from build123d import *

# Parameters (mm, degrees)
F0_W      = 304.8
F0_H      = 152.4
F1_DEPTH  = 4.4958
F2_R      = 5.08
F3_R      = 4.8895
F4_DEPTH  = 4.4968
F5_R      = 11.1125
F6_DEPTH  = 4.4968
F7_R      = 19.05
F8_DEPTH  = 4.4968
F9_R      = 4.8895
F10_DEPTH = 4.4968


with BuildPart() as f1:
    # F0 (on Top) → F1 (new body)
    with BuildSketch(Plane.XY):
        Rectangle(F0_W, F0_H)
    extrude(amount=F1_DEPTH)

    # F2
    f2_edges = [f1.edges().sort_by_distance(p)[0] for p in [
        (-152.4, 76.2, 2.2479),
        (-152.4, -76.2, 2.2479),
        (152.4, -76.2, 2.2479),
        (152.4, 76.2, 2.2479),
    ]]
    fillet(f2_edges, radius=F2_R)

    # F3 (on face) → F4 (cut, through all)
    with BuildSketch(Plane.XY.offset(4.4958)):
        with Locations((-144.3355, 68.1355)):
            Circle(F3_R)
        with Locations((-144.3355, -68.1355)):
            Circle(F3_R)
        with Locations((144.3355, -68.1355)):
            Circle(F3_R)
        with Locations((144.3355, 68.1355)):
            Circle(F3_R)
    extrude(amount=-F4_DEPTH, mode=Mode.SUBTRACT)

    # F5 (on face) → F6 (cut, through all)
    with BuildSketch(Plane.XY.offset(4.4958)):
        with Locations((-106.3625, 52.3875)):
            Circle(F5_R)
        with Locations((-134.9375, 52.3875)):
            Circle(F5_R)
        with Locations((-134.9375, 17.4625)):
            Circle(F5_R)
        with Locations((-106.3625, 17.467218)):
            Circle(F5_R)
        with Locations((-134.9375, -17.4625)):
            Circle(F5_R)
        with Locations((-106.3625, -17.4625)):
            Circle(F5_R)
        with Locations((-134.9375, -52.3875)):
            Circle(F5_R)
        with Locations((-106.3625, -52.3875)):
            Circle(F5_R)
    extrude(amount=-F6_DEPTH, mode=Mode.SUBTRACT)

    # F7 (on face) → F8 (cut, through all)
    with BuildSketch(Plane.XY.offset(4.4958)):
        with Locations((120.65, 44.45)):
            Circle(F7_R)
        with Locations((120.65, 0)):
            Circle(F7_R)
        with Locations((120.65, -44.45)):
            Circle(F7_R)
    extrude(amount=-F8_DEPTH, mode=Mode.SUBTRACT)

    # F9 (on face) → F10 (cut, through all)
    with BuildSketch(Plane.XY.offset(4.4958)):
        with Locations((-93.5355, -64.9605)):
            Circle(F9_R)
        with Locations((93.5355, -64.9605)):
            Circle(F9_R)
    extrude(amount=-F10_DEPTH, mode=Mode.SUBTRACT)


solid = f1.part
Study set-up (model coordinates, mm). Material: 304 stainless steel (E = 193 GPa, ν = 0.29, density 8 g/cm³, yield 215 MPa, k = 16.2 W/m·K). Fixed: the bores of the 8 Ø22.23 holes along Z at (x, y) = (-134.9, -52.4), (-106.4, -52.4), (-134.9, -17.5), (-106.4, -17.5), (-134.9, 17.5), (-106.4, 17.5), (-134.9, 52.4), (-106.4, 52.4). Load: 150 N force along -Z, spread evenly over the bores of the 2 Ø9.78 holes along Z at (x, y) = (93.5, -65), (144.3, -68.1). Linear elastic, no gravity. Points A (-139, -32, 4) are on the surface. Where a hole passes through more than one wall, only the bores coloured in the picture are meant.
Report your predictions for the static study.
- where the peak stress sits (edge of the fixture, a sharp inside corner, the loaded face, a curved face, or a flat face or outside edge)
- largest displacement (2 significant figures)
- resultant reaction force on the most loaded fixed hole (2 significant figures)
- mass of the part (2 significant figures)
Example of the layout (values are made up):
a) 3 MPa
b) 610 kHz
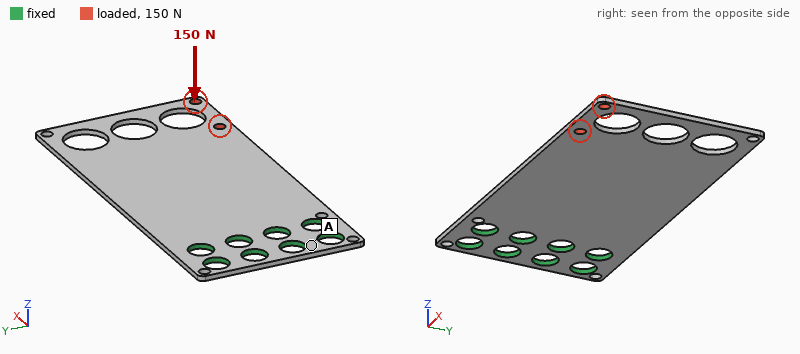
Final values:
a) a curved face
b) 3.2 mm
c) 91 N
d) 1.4 kg
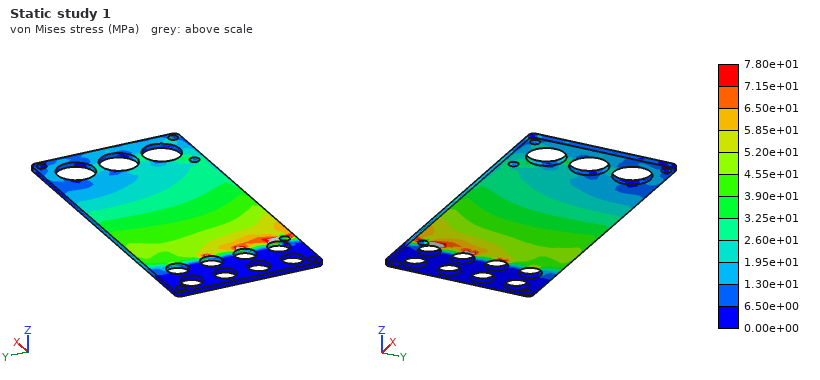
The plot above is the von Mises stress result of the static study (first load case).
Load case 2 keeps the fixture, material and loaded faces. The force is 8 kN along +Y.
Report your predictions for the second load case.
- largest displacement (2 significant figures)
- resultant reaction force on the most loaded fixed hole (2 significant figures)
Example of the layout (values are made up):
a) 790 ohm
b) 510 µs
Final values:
a) 0.25 mm
b) 14 kN
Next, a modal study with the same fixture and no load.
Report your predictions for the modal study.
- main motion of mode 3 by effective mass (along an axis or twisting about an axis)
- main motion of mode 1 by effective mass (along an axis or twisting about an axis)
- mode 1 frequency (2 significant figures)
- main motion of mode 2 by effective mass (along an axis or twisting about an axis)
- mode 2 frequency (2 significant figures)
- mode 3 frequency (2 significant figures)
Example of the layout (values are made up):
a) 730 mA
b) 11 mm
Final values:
a) along Z
b) along Z
c) 68 Hz
d) twisting about X
e) 230 Hz
f) 370 Hz
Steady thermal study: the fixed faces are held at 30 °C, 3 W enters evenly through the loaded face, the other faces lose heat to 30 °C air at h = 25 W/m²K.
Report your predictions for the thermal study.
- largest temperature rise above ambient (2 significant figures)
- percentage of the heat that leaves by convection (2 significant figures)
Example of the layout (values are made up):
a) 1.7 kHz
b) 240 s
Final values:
a) 30 K
b) 100 %
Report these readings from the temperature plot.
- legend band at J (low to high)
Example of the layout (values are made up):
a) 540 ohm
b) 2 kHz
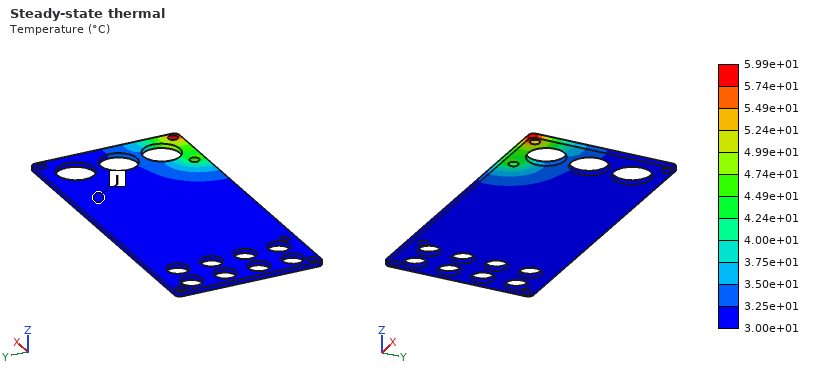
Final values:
a) 3.00e+01 to 3.25e+01 °C
